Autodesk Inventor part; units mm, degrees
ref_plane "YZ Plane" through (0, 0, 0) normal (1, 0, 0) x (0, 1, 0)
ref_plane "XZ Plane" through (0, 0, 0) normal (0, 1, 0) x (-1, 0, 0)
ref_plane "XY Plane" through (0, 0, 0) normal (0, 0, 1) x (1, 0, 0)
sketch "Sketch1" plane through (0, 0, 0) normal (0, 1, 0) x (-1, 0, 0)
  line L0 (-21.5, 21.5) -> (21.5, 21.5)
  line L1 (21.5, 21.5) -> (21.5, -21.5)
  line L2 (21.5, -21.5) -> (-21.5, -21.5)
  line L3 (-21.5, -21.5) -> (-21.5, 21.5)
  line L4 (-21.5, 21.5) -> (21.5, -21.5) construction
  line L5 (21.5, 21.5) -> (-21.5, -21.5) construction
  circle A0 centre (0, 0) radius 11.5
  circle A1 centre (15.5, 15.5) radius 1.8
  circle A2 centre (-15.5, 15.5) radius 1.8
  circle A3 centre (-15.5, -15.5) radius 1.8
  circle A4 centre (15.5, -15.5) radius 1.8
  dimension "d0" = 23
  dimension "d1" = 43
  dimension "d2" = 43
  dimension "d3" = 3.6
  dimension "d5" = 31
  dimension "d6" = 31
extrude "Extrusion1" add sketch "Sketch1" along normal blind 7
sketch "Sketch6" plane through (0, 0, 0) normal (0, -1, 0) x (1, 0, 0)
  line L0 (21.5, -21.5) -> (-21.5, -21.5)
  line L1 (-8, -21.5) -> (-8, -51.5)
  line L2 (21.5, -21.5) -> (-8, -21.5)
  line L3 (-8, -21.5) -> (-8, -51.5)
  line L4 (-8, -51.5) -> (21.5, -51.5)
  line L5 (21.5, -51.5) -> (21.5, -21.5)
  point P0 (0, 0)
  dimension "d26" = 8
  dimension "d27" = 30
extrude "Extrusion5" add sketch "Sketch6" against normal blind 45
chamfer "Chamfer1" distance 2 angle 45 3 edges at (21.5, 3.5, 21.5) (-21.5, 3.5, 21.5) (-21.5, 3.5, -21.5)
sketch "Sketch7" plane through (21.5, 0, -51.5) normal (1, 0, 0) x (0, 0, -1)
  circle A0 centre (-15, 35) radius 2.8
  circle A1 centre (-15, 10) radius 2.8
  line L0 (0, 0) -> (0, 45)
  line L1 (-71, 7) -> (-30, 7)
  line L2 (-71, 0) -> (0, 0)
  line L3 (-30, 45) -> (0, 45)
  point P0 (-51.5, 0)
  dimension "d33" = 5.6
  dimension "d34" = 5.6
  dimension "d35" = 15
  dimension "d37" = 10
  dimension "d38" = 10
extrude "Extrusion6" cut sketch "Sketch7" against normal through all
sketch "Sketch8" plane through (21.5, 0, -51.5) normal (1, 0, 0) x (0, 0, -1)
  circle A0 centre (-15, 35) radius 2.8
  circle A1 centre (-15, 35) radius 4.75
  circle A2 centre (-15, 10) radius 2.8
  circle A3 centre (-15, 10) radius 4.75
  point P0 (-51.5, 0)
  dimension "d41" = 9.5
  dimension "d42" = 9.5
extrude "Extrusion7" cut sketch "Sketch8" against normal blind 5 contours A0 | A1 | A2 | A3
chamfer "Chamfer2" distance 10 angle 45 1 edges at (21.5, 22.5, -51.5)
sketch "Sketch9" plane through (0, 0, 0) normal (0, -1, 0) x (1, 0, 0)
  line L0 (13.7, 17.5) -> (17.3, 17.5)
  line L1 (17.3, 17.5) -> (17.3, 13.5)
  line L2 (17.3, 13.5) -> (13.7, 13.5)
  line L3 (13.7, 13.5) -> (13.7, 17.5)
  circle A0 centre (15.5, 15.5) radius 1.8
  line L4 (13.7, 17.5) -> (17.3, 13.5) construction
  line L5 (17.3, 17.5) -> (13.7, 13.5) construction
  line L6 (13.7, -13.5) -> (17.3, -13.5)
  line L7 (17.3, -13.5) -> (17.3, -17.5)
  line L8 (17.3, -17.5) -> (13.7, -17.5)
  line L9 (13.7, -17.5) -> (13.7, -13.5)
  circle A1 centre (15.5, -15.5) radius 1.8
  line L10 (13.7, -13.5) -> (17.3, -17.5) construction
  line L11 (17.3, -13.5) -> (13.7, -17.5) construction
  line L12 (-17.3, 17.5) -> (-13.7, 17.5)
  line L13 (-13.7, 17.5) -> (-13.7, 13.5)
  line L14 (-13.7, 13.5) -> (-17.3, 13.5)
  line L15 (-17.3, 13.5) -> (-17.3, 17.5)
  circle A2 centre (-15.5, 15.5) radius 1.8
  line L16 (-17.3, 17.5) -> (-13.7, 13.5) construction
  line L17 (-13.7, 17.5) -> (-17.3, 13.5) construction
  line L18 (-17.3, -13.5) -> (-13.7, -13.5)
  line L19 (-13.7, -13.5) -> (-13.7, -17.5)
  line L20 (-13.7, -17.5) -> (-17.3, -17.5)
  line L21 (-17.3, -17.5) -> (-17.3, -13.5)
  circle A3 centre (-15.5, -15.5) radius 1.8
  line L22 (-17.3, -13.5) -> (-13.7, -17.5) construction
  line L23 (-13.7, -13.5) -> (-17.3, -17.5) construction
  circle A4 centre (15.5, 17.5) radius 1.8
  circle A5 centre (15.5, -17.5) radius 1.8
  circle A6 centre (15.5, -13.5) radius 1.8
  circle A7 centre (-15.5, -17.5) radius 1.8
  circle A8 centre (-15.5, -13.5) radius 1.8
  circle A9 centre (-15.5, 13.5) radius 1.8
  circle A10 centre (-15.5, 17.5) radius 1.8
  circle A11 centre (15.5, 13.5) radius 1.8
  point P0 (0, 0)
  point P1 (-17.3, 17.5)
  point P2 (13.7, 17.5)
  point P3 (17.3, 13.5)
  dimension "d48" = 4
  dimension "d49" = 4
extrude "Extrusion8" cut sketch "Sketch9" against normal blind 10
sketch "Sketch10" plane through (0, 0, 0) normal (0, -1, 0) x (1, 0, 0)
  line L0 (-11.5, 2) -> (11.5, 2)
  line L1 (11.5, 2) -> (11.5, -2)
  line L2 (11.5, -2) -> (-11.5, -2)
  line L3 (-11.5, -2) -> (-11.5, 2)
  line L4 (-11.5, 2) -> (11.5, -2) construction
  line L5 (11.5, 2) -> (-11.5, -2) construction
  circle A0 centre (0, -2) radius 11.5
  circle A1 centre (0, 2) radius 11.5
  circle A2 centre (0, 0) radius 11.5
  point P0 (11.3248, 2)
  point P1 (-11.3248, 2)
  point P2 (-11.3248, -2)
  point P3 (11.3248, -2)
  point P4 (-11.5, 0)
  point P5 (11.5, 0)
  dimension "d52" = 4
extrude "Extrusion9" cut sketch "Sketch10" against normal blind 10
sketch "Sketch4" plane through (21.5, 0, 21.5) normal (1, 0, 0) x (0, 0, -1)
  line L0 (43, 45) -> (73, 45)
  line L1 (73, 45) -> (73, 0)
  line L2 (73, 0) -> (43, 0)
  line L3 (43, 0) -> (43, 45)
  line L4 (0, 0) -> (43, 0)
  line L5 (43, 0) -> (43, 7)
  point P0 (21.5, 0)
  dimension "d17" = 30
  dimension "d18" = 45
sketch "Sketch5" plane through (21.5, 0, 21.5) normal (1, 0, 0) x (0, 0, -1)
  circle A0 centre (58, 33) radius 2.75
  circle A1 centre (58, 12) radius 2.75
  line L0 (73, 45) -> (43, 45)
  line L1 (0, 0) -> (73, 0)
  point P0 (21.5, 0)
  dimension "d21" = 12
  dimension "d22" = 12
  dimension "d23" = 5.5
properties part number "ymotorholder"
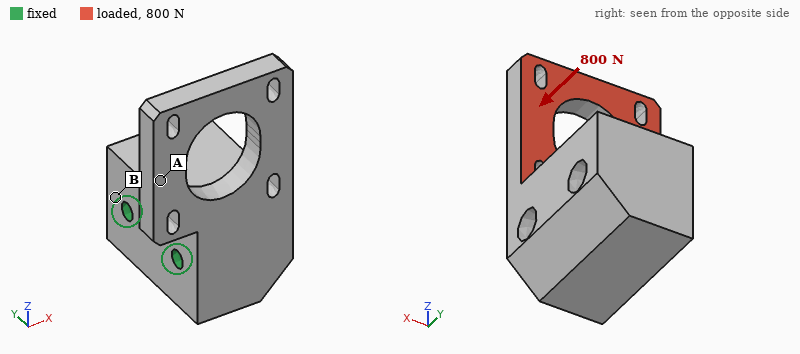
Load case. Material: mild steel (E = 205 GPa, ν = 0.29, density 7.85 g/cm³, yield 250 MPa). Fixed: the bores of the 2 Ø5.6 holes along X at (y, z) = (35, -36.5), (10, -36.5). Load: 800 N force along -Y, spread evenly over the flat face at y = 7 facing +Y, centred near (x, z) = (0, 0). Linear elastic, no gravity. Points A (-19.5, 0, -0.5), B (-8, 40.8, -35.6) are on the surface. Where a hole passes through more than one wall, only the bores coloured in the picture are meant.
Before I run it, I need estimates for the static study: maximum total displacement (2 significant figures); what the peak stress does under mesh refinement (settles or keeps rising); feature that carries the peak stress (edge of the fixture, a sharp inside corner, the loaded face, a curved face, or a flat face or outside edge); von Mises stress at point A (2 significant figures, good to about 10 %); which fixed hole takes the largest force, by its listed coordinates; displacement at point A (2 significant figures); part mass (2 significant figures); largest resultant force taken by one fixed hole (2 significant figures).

0.11 mm
keeps rising
a sharp inside corner
22 MPa
(35, -36.5)
0.048 mm
350 g
1.1 kN
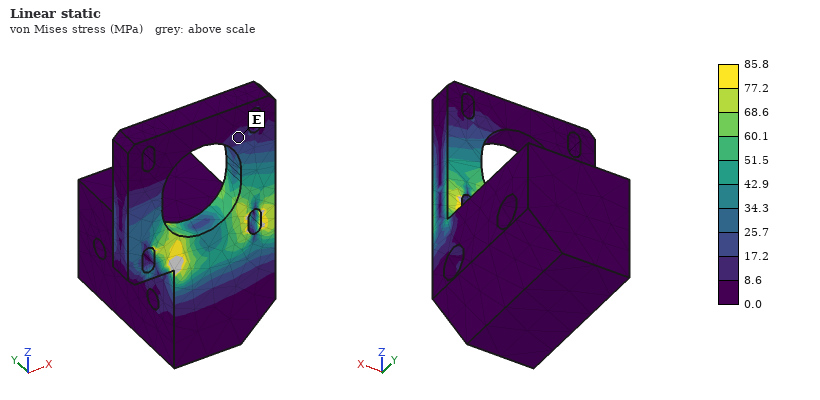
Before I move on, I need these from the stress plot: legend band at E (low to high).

8.6 to 17.2 MPa
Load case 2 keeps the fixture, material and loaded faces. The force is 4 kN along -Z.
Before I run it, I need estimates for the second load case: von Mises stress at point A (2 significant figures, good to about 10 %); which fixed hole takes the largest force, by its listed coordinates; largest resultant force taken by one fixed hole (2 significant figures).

46 MPa
(10, -36.5)
4.2 kN
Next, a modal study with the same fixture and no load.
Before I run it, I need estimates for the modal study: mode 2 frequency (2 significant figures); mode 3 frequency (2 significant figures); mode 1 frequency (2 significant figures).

4400 Hz
4700 Hz
2100 Hz
